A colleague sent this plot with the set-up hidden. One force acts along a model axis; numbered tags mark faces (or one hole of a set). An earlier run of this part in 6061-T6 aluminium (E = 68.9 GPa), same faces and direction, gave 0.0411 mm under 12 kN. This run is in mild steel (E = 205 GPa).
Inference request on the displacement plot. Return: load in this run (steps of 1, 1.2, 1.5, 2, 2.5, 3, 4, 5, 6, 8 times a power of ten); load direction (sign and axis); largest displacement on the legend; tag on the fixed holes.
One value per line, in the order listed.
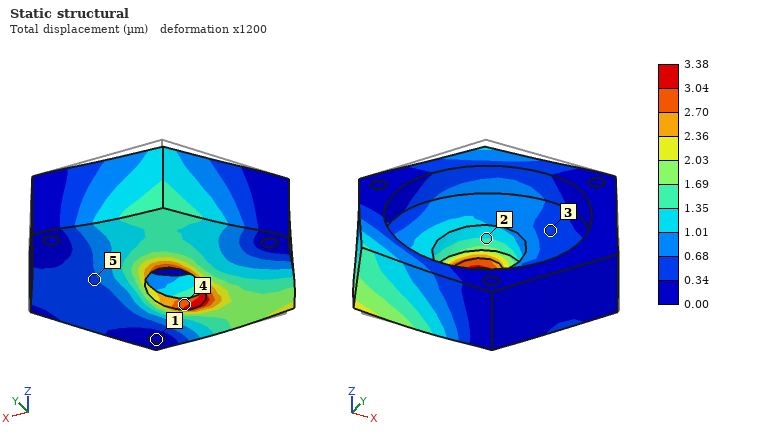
3 kN
-Y
3.38 µm
1
